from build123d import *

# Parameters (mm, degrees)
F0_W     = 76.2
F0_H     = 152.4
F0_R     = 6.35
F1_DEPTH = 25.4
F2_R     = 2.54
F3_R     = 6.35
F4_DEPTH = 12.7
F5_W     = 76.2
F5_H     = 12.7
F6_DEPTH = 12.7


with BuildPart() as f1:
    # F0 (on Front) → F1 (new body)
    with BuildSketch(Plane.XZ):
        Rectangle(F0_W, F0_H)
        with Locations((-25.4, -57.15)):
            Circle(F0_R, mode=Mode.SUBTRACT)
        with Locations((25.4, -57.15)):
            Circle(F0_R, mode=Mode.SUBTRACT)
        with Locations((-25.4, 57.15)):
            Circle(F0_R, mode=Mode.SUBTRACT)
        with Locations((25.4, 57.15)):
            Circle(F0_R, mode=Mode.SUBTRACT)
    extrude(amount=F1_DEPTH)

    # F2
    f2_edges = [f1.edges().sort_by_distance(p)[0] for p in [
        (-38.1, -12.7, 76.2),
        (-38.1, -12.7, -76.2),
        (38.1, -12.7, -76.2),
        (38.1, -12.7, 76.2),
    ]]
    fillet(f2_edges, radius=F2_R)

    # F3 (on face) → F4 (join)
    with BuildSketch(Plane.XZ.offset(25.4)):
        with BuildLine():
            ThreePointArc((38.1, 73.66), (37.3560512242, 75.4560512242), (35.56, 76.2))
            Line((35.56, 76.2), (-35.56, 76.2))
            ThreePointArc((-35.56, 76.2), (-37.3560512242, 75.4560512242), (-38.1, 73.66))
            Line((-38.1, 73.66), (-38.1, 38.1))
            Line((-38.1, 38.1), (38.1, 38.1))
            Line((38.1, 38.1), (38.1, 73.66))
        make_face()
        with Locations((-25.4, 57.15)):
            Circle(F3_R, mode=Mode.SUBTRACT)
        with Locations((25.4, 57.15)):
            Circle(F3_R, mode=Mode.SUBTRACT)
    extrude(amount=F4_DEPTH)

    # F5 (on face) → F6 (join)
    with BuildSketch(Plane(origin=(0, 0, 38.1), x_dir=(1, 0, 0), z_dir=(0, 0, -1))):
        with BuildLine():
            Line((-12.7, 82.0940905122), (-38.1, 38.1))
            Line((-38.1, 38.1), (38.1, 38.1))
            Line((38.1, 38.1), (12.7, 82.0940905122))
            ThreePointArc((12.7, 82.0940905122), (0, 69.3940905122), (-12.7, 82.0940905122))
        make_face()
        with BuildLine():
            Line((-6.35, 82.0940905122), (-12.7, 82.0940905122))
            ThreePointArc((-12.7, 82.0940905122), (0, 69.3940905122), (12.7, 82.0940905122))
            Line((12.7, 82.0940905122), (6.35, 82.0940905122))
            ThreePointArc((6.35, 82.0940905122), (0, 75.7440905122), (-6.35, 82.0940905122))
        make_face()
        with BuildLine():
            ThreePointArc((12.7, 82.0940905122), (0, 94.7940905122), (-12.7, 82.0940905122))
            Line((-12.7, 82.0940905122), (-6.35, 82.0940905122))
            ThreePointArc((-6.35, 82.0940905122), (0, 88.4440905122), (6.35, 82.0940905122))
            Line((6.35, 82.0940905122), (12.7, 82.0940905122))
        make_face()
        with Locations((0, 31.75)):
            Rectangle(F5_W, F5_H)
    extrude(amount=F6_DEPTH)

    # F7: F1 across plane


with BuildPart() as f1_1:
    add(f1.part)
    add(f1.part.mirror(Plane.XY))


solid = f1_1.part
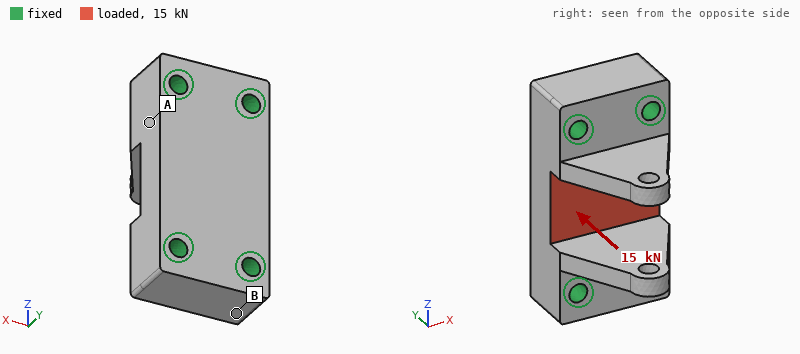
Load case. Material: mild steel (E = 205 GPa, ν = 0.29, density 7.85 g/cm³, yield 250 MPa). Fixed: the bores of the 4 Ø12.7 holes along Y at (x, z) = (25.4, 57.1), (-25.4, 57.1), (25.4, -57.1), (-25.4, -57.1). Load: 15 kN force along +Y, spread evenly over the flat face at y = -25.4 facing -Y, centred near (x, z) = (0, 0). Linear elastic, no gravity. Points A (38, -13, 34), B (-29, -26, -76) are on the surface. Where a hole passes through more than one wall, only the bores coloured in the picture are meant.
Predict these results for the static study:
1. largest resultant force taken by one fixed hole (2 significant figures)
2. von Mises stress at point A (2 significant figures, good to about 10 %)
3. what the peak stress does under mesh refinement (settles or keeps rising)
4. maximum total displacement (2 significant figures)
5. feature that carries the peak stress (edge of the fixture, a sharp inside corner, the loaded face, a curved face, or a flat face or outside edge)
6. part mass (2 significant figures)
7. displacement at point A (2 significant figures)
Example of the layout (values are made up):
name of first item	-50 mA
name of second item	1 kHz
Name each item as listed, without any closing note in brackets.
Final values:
largest resultant force taken by one fixed hole	3.9 kN
von Mises stress at point A	7.9 MPa
what the peak stress does under mesh refinement	keeps rising
maximum total displacement	5.2 µm
feature that carries the peak stress	edge of the fixture
part mass	3.4 kg
displacement at point A	1.4 µm
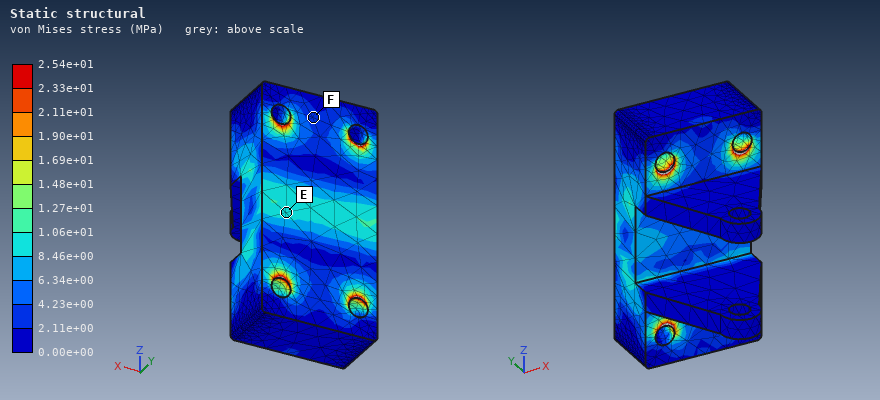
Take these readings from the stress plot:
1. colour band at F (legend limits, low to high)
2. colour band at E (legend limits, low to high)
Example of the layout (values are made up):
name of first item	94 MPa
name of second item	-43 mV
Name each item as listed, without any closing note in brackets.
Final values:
colour band at F	2.11e+00 to 4.23e+00 MPa
colour band at E	8.46e+00 to 1.06e+01 MPa
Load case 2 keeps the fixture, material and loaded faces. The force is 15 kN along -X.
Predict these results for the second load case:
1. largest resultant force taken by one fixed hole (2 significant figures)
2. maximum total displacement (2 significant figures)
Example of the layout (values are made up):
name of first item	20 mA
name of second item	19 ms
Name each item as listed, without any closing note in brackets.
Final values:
largest resultant force taken by one fixed hole	5.0 kN
maximum total displacement	4.1 µm
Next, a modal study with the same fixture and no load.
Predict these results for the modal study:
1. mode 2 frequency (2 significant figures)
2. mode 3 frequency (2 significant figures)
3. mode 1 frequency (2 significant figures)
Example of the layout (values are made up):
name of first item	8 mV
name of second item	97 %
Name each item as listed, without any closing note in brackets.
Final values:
mode 2 frequency	4200 Hz
mode 3 frequency	9500 Hz
mode 1 frequency	4200 Hz
